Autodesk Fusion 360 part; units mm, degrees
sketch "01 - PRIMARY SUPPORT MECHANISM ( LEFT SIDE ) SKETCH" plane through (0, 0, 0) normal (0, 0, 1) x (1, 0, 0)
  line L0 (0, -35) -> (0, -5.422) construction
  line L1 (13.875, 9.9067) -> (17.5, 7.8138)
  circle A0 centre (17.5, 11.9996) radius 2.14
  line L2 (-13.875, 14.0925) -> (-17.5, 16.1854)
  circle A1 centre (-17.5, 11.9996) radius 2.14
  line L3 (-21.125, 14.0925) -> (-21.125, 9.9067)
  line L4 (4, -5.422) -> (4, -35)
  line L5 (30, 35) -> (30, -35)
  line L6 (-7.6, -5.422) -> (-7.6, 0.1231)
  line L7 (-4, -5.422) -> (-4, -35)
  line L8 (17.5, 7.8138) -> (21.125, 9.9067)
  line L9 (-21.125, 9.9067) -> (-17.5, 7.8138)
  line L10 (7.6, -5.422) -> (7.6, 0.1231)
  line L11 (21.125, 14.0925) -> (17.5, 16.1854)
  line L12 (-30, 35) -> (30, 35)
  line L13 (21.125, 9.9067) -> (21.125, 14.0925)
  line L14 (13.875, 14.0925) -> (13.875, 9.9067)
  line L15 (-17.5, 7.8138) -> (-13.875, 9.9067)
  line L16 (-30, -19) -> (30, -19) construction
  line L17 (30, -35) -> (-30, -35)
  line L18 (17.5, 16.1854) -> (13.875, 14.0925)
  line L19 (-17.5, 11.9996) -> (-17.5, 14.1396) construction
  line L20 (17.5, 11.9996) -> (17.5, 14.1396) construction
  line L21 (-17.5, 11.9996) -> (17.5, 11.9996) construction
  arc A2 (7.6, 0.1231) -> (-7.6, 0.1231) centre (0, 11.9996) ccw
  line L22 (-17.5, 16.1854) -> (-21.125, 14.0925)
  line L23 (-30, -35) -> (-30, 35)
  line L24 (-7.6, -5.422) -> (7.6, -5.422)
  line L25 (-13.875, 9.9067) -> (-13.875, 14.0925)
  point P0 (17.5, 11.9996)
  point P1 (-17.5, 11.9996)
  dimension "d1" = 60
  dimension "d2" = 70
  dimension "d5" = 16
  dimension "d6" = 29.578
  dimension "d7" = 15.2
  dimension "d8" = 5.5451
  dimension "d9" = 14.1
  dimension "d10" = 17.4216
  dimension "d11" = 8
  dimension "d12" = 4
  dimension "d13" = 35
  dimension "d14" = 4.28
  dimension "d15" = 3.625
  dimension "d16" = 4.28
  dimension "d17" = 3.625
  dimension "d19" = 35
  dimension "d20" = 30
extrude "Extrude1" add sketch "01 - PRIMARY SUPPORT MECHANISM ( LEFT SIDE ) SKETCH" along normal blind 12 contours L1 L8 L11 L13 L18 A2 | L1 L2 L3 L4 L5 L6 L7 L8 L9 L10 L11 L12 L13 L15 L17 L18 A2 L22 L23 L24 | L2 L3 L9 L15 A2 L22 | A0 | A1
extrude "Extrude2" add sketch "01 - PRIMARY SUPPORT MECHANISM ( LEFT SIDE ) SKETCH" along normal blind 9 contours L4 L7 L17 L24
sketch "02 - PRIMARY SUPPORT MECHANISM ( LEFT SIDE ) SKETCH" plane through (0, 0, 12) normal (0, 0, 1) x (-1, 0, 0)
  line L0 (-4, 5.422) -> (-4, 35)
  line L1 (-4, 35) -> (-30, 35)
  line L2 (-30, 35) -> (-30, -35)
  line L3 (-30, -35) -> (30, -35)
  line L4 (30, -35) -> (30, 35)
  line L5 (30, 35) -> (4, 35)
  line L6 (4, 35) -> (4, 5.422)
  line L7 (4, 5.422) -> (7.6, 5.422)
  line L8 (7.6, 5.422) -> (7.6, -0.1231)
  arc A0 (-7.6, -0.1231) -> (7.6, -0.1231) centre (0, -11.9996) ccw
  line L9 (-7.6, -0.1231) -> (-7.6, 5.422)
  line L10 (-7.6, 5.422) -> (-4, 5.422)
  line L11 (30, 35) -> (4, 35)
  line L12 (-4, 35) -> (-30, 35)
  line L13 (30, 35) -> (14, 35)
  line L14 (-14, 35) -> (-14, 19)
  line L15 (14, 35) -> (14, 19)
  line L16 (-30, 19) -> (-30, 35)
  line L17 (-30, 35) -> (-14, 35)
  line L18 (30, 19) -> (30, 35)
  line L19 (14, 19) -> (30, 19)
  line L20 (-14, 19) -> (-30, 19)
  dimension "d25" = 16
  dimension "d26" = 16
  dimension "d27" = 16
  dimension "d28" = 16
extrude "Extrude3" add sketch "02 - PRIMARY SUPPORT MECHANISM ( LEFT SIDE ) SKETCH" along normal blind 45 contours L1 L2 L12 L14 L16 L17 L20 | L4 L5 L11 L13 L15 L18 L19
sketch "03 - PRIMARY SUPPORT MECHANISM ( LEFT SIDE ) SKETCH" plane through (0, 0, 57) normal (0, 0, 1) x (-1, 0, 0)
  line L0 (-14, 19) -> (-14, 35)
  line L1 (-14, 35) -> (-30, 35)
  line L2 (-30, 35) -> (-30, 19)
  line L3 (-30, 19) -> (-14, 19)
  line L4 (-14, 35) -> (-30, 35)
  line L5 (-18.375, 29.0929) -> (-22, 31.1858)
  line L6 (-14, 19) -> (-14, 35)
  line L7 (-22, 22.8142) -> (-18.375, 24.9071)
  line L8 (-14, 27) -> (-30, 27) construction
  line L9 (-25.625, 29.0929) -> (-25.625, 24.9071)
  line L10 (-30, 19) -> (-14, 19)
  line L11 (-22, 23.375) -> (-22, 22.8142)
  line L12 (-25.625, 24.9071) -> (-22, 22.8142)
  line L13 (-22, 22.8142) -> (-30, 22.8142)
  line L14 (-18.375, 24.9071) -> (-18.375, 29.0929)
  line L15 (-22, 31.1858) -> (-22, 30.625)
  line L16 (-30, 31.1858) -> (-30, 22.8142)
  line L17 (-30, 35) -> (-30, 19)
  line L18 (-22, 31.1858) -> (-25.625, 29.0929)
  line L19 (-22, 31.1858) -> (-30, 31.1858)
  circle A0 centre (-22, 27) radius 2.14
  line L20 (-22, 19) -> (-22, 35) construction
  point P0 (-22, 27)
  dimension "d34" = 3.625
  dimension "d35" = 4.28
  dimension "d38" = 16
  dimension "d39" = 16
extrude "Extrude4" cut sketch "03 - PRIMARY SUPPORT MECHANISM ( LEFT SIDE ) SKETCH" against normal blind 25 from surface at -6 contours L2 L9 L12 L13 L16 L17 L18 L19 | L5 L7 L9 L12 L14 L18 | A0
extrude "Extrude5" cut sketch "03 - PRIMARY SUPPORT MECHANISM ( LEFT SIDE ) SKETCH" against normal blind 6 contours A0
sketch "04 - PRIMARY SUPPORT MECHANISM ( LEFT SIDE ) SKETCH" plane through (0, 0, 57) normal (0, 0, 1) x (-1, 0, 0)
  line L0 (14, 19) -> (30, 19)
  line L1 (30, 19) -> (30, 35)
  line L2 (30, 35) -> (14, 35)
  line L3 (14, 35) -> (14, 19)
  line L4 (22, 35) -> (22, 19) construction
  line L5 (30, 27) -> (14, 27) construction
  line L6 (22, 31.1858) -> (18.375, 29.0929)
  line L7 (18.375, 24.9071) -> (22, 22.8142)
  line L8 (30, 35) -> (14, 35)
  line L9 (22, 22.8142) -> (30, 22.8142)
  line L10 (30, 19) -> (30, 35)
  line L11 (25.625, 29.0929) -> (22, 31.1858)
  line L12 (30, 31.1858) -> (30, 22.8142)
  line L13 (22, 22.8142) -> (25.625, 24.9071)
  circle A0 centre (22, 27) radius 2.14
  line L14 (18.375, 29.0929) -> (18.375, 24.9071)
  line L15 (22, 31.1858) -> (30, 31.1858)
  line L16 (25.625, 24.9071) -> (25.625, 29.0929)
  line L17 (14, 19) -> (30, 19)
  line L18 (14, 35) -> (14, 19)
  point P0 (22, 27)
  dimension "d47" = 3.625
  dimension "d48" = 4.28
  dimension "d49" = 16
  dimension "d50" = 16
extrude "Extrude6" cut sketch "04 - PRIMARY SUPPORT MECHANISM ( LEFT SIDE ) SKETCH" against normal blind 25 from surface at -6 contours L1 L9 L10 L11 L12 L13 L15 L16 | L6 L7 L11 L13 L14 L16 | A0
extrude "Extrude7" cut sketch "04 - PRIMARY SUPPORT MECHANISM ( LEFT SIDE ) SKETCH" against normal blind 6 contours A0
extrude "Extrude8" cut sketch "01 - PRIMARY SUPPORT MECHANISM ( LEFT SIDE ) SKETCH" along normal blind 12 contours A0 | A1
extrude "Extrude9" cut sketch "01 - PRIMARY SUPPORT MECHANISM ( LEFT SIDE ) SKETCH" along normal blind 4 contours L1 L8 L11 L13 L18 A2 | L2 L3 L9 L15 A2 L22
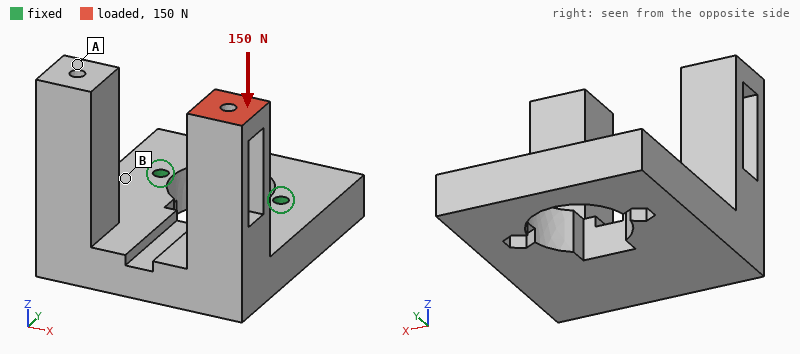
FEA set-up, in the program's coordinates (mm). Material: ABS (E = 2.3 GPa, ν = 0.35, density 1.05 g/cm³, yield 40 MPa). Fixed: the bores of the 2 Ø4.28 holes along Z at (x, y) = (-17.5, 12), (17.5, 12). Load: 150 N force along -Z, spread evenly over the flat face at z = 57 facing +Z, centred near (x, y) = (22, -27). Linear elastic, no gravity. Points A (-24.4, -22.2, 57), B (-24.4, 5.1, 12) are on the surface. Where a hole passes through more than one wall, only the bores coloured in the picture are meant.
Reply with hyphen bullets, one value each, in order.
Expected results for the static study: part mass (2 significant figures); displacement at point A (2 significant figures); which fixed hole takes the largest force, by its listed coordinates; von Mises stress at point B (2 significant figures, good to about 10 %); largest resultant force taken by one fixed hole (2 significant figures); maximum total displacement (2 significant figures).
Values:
- 62 g
- 0.68 mm
- (17.5, 12)
- 4.2 MPa
- 140 N
- 1.2 mm
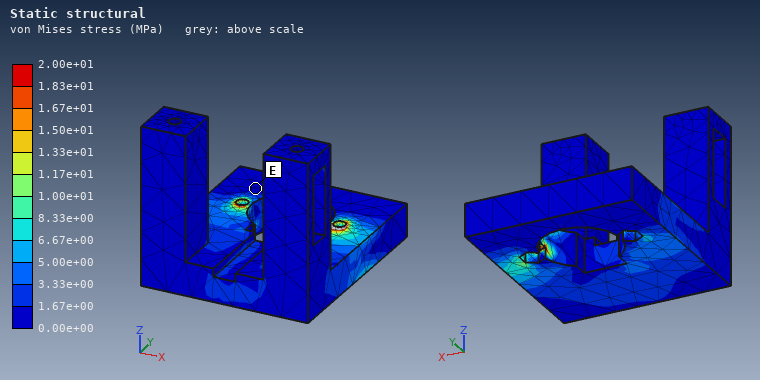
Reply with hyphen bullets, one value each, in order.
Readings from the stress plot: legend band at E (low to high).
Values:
- 0.00e+00 to 1.67e+00 MPa
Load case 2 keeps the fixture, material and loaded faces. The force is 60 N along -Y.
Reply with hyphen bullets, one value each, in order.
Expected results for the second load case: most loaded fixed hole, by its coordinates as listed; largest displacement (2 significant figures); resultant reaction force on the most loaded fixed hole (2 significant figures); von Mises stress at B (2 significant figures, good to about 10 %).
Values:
- (17.5, 12)
- 1.1 mm
- 68 N
- 2.9 MPa
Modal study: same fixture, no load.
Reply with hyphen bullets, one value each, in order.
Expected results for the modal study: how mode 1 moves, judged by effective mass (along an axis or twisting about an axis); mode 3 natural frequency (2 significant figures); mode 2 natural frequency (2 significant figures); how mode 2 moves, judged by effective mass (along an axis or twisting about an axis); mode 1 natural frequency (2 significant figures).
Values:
- along Z
- 890 Hz
- 610 Hz
- along X
- 390 Hz
